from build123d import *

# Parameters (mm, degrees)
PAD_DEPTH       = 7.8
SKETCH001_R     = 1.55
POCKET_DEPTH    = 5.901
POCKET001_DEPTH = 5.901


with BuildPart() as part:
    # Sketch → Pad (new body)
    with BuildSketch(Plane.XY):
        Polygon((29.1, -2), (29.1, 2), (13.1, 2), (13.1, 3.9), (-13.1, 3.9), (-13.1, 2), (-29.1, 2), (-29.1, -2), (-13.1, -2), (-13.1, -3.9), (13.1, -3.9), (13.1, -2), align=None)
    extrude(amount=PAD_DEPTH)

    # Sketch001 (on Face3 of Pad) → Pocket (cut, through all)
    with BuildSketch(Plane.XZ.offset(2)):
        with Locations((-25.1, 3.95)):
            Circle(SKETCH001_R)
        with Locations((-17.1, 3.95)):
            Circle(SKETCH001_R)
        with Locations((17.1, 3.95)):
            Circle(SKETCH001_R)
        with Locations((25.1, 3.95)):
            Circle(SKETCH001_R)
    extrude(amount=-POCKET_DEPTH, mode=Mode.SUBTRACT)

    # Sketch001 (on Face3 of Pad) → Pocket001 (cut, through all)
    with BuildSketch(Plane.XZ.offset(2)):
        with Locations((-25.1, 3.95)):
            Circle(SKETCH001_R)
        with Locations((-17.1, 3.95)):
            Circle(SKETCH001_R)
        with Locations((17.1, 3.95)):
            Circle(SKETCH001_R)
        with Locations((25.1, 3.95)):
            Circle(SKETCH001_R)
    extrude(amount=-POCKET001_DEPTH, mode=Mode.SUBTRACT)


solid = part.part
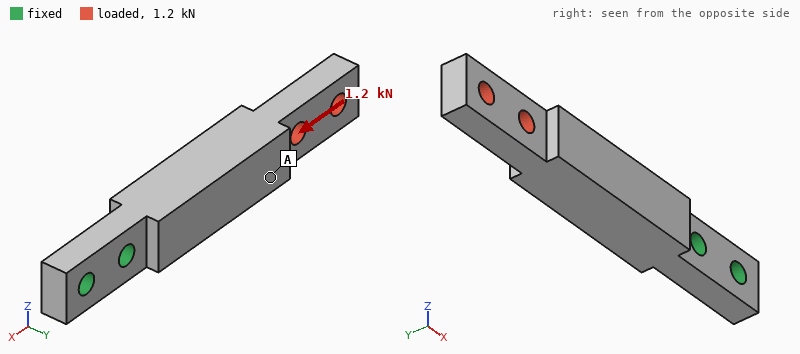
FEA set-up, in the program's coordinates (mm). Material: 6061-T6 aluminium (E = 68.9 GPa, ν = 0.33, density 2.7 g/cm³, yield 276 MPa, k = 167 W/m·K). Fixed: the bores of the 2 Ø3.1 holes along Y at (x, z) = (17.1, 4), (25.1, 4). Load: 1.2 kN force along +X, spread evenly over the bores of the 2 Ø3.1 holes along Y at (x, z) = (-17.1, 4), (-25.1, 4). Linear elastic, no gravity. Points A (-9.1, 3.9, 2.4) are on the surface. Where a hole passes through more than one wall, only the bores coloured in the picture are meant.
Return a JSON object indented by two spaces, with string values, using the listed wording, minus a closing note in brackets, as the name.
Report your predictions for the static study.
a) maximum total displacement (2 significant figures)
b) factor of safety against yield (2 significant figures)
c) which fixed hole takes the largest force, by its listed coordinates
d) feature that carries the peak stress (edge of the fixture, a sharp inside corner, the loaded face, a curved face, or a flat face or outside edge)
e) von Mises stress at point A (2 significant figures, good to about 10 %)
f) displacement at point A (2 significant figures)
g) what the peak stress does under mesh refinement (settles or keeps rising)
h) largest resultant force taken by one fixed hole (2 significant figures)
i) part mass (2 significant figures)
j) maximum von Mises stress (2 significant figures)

{
  "maximum total displacement": "18 µm",
  "factor of safety against yield": "2.5",
  "which fixed hole takes the largest force, by its listed coordinates": "(17.1, 4)",
  "feature that carries the peak stress": "the loaded face",
  "von Mises stress at point A": "14 MPa",
  "displacement at point A": "8.8 µm",
  "what the peak stress does under mesh refinement": "settles",
  "largest resultant force taken by one fixed hole": "1.1 kN",
  "part mass": "6.7 g",
  "maximum von Mises stress": "110 MPa"
}
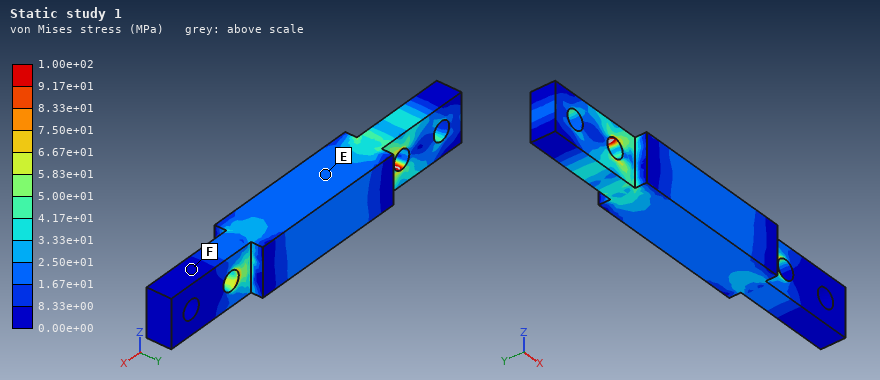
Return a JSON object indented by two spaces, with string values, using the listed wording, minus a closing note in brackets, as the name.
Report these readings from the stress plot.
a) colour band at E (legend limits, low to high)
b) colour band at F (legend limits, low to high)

{
  "colour band at E": "1.67e+01 to 2.50e+01 MPa",
  "colour band at F": "0.00e+00 to 8.33e+00 MPa"
}
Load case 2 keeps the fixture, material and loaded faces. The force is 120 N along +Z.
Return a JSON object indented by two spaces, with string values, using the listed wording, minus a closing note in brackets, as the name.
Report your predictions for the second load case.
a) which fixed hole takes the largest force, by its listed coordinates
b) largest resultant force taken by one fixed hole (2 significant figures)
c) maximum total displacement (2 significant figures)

{
  "which fixed hole takes the largest force, by its listed coordinates": "(17.1, 4)",
  "largest resultant force taken by one fixed hole": "310 N",
  "maximum total displacement": "0.22 mm"
}
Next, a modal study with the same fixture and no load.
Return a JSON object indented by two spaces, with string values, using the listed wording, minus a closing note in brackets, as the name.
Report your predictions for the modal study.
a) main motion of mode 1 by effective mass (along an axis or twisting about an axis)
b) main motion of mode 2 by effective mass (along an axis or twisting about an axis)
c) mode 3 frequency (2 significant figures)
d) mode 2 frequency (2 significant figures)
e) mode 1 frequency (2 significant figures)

{
  "main motion of mode 1 by effective mass": "along Y",
  "main motion of mode 2 by effective mass": "along Z",
  "mode 3 frequency": "12 kHz",
  "mode 2 frequency": "3100 Hz",
  "mode 1 frequency": "2200 Hz"
}
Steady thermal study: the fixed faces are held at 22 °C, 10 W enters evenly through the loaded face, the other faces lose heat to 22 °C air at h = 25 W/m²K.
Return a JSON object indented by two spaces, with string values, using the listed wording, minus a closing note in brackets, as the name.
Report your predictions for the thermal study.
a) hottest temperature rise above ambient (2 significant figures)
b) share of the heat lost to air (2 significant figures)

{
  "hottest temperature rise above ambient": "51 K",
  "share of the heat lost to air": "8.3 %"
}
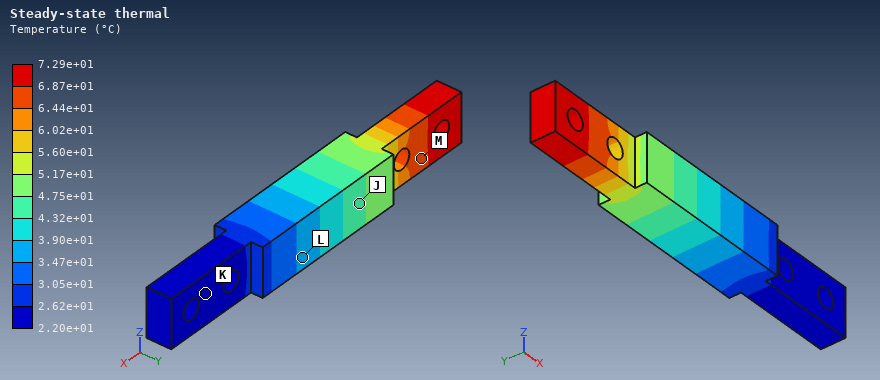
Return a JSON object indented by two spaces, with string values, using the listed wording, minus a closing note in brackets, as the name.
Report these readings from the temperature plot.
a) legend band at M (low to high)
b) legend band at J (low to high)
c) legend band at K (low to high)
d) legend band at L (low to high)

{
  "legend band at M": "6.44e+01 to 6.87e+01 °C",
  "legend band at J": "4.32e+01 to 4.75e+01 °C",
  "legend band at K": "2.20e+01 to 2.62e+01 °C",
  "legend band at L": "3.47e+01 to 3.90e+01 °C"
}
